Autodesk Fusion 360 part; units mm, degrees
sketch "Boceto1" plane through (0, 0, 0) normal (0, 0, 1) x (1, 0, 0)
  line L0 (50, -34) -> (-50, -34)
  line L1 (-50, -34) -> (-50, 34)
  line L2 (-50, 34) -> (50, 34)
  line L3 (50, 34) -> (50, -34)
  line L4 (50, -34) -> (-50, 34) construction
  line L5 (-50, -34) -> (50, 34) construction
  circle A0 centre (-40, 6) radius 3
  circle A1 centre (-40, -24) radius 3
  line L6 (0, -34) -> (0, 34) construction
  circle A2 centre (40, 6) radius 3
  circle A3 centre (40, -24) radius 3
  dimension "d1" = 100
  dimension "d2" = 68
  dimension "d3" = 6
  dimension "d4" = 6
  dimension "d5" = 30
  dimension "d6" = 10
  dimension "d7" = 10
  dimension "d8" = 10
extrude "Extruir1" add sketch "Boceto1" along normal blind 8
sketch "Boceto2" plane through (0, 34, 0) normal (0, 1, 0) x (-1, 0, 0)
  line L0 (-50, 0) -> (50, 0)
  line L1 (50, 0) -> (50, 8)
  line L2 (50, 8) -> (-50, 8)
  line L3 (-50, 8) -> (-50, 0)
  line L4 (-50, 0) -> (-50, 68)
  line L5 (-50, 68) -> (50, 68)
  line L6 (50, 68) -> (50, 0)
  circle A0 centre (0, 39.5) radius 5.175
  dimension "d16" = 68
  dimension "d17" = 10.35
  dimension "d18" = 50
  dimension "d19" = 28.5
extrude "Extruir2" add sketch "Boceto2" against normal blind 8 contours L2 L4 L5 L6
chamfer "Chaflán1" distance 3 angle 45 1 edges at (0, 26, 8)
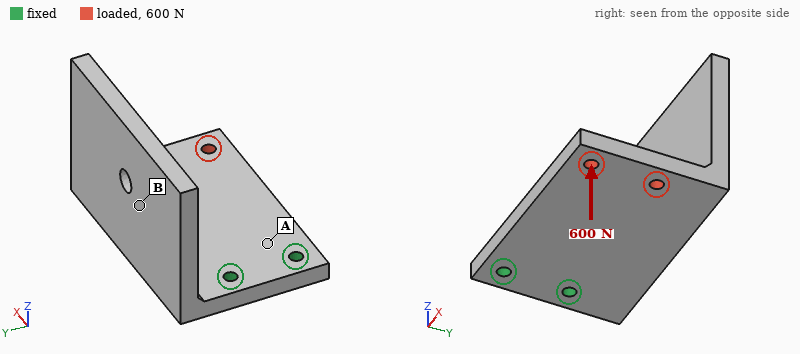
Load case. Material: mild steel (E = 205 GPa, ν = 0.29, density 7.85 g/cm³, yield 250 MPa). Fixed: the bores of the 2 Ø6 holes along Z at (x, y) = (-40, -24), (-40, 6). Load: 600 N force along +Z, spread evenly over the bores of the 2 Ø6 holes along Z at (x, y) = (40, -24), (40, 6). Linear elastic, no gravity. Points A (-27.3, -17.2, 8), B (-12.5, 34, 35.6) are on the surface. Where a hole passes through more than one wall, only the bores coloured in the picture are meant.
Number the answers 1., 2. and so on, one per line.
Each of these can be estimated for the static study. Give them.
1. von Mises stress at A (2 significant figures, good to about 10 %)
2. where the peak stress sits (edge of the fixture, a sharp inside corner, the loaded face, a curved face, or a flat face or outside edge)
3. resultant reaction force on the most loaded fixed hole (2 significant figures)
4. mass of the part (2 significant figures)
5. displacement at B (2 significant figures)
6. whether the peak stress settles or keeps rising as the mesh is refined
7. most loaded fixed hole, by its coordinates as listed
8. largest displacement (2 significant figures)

1. 40 MPa
2. edge of the fixture
3. 380 N
4. 790 g
5. 0.053 mm
6. keeps rising
7. (-40, 6)
8. 0.15 mm
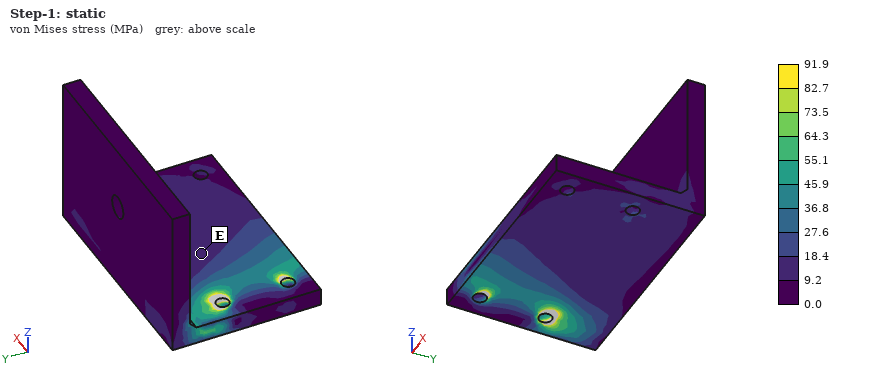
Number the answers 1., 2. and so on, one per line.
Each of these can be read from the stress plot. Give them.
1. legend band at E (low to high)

1. 9.2 to 18.4 MPa
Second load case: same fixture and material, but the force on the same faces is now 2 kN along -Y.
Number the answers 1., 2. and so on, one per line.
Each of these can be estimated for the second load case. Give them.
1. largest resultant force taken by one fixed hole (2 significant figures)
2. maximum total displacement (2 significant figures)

1. 4.8 kN
2. 26 µm
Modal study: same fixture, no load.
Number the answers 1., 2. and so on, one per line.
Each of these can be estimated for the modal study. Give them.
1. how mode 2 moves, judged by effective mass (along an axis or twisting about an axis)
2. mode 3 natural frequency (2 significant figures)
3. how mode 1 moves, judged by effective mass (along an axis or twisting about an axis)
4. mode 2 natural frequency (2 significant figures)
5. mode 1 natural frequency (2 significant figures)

1. along Y
2. 2100 Hz
3. along Z
4. 880 Hz
5. 550 Hz
